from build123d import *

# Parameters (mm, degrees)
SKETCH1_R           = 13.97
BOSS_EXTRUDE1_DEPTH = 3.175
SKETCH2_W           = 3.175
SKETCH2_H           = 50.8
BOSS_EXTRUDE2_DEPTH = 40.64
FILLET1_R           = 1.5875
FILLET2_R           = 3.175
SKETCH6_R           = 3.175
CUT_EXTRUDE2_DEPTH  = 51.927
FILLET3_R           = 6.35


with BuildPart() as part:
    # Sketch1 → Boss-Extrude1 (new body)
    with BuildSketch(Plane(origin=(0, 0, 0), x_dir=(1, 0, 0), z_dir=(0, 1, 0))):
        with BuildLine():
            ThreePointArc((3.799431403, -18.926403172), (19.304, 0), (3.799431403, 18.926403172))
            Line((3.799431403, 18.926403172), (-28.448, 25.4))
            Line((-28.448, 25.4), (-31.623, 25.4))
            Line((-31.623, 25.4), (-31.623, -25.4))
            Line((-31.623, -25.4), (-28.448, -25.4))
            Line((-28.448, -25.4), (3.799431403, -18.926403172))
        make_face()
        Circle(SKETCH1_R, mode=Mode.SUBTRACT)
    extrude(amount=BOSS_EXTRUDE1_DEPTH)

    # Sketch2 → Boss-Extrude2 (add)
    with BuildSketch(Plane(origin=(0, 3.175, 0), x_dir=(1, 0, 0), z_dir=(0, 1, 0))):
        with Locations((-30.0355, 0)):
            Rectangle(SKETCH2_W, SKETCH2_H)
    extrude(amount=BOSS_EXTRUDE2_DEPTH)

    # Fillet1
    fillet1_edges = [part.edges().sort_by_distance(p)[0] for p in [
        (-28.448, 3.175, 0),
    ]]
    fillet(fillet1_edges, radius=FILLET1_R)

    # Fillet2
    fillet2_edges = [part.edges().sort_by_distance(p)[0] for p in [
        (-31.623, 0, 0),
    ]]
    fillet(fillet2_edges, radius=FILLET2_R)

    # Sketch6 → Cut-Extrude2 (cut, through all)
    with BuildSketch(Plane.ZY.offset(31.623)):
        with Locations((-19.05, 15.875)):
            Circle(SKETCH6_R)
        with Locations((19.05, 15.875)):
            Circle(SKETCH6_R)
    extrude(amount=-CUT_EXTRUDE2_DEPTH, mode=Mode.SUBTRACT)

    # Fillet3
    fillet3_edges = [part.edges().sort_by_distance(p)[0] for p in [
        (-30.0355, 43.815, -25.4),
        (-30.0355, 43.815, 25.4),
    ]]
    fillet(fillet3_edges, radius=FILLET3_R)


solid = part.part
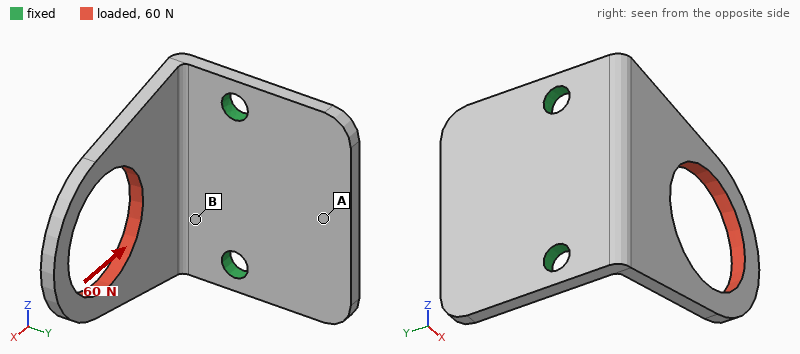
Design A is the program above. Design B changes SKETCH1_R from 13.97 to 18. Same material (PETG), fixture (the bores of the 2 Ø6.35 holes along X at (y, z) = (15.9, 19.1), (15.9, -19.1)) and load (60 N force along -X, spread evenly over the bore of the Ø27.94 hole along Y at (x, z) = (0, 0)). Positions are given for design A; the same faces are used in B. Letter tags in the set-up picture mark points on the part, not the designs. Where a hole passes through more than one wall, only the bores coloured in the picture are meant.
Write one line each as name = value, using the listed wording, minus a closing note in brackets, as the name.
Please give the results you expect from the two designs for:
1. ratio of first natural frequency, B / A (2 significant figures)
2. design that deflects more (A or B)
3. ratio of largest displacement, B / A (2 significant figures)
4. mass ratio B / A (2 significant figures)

ratio of first natural frequency, B / A = 1.4
design that deflects more = B
ratio of largest displacement, B / A = 1.3
mass ratio B / A = 0.88
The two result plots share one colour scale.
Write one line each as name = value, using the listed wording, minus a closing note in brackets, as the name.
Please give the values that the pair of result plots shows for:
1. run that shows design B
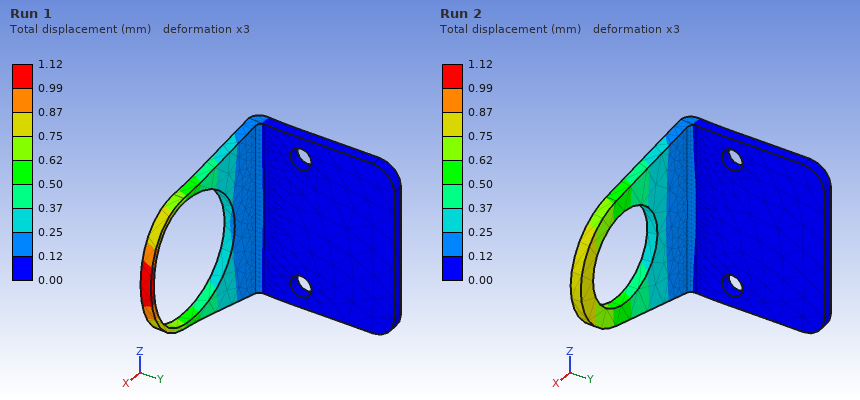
run that shows design B = Run 1
